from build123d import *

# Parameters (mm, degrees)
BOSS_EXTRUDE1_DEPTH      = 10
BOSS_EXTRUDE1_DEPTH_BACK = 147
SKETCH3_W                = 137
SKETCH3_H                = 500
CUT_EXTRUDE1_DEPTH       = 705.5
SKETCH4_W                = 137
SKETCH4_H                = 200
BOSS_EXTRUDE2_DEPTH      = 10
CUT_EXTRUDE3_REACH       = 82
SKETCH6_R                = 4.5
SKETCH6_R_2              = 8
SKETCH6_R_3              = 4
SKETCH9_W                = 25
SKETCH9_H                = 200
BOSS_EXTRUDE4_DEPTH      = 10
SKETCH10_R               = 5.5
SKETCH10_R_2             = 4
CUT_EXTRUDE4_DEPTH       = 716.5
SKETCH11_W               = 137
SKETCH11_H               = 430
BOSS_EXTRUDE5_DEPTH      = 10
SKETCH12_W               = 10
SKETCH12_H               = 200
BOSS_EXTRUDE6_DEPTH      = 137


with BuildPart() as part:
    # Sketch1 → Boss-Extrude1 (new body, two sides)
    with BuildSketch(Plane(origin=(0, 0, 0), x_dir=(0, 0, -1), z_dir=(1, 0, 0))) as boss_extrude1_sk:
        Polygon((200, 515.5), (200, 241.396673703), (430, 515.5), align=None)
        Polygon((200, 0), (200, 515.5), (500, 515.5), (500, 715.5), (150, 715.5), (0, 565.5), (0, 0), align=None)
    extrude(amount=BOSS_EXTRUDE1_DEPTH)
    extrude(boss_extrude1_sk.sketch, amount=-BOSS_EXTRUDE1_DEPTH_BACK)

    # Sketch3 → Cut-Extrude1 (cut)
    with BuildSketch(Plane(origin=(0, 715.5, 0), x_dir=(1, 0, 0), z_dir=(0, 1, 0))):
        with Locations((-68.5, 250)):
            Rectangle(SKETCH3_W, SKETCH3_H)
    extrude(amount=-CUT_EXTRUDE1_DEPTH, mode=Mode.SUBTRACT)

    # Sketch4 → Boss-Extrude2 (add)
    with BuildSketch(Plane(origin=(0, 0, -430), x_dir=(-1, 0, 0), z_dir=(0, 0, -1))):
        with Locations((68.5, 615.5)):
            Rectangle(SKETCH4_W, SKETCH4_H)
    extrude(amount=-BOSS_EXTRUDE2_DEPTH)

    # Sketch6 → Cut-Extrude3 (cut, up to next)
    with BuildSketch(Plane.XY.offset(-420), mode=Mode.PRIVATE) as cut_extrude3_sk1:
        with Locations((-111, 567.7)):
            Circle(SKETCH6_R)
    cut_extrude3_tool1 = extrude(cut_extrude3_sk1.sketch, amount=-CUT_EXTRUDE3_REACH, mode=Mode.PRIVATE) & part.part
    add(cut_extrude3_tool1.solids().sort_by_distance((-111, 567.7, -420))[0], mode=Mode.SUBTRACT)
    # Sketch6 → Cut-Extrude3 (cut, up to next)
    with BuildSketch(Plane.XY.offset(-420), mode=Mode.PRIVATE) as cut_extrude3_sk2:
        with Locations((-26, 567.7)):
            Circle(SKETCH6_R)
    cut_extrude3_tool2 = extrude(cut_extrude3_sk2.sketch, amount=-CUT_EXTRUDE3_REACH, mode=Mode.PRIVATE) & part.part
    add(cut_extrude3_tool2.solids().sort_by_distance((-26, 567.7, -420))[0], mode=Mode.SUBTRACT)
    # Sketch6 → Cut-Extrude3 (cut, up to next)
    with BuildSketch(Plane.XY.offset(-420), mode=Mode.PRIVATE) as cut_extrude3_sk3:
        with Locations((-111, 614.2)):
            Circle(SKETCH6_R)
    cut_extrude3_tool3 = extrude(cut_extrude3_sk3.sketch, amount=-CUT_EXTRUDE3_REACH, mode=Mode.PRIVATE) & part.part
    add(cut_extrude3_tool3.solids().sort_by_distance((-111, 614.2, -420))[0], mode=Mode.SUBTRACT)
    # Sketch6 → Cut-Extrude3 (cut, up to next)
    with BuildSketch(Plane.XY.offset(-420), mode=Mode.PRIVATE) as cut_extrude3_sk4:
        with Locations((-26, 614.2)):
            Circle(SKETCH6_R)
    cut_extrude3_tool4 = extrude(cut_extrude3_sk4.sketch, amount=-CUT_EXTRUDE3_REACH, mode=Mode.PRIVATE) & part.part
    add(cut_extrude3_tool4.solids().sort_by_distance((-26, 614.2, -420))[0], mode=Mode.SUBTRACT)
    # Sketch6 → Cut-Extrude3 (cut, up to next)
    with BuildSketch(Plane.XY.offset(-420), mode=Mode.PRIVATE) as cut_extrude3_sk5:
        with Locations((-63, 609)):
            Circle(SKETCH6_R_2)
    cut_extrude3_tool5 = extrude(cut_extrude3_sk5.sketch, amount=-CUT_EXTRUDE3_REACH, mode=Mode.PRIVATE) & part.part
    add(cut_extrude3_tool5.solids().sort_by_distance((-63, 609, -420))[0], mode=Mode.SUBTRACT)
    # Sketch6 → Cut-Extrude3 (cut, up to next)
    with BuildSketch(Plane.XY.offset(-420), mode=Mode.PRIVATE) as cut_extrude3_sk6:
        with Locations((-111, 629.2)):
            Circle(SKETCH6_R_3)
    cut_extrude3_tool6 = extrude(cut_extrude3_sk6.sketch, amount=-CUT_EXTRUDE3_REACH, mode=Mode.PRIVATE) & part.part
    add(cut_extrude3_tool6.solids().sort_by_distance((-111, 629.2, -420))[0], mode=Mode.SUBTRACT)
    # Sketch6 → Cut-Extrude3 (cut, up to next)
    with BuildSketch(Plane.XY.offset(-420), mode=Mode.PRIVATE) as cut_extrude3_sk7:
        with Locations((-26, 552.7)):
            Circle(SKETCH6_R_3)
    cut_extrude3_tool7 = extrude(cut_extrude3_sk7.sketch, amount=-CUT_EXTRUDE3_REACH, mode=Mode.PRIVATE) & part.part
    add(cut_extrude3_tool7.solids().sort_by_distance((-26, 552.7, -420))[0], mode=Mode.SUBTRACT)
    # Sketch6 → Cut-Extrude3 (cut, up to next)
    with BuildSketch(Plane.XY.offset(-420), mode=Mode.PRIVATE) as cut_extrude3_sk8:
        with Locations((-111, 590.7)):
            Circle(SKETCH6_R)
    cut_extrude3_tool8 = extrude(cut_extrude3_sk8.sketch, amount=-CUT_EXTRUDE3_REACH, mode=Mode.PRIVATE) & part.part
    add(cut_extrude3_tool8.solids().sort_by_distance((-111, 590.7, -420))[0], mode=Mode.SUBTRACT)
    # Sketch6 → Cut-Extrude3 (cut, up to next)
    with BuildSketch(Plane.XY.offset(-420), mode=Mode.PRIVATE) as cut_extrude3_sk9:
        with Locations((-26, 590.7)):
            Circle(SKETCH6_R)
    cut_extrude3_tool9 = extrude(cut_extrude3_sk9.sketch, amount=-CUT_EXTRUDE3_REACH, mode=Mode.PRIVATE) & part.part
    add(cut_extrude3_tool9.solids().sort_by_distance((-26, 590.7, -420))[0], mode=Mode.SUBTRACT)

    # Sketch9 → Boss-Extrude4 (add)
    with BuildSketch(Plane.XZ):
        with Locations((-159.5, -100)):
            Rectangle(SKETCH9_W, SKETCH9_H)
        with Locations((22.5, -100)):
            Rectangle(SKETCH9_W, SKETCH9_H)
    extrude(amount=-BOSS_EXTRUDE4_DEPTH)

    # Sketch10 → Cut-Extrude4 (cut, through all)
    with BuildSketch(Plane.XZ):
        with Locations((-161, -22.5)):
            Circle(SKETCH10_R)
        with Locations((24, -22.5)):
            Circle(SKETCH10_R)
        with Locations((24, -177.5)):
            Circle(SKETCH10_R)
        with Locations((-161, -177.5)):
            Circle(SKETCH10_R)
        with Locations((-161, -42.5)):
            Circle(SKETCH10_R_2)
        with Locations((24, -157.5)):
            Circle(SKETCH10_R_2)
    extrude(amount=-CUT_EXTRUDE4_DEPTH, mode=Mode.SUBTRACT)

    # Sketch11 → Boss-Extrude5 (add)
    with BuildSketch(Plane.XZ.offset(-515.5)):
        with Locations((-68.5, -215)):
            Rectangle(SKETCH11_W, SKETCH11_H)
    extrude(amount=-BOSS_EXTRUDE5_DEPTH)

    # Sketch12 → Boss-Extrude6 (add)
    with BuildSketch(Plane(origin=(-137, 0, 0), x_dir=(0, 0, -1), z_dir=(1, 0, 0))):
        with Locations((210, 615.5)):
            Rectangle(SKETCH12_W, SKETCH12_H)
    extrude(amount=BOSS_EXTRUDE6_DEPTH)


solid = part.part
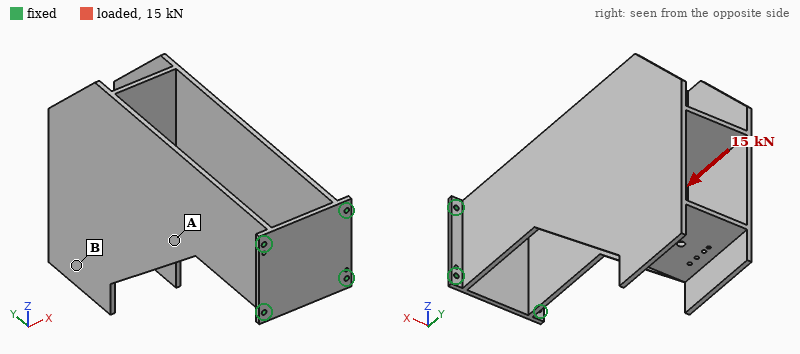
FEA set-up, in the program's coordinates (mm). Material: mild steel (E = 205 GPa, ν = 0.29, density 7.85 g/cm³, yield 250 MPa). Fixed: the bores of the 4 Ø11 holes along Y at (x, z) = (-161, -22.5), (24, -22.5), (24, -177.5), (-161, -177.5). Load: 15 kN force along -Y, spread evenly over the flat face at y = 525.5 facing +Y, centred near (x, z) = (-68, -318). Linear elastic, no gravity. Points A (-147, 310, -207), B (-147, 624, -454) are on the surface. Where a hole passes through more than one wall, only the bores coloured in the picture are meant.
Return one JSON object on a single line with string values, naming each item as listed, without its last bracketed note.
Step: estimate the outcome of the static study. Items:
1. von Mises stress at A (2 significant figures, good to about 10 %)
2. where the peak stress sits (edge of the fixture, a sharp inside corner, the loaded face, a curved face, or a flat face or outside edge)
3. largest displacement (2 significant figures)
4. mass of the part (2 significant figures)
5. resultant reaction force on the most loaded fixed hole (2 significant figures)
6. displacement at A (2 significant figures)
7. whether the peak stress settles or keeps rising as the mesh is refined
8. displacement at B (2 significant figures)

{"von Mises stress at A": "12 MPa", "where the peak stress sits": "edge of the fixture", "largest displacement": "0.51 mm", "mass of the part": "47 kg", "resultant reaction force on the most loaded fixed hole": "14 kN", "displacement at A": "0.16 mm", "whether the peak stress settles or keeps rising as the mesh is refined": "keeps rising", "displacement at B": "0.44 mm"}
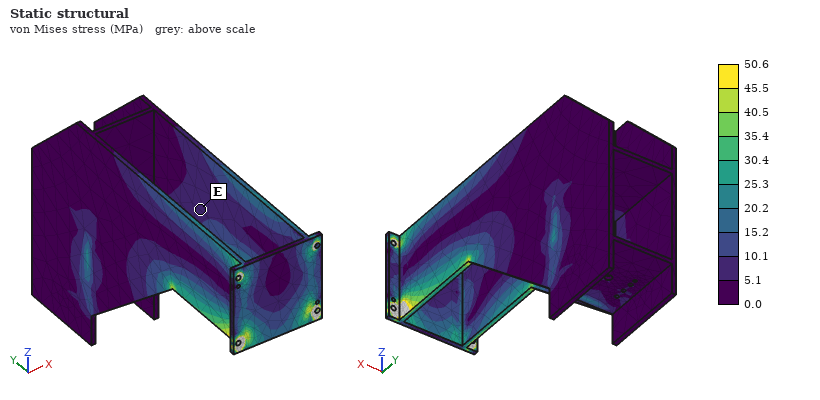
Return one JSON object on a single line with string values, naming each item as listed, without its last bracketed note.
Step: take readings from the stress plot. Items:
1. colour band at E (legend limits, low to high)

{"colour band at E": "5.1 to 10.1 MPa"}
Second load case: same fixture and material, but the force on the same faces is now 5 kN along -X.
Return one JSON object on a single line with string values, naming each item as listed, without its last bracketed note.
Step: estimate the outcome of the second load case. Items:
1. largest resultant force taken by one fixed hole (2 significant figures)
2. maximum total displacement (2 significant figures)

{"largest resultant force taken by one fixed hole": "16 kN", "maximum total displacement": "7.6 mm"}
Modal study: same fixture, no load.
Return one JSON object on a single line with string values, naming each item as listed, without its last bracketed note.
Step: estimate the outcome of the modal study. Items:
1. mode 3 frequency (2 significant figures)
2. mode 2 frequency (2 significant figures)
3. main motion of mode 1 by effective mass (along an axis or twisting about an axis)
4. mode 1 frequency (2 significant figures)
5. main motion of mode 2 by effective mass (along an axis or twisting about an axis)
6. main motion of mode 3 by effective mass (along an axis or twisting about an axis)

{"mode 3 frequency": "120 Hz", "mode 2 frequency": "100 Hz", "main motion of mode 1 by effective mass": "along X", "mode 1 frequency": "24 Hz", "main motion of mode 2 by effective mass": "twisting about Y", "main motion of mode 3 by effective mass": "along Z"}
